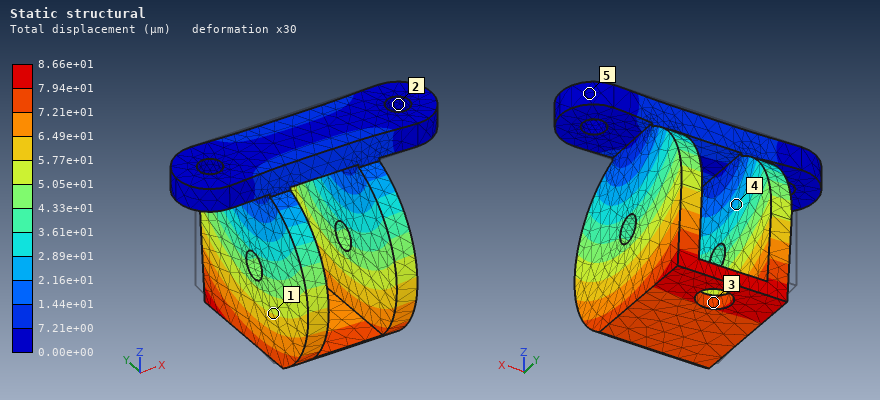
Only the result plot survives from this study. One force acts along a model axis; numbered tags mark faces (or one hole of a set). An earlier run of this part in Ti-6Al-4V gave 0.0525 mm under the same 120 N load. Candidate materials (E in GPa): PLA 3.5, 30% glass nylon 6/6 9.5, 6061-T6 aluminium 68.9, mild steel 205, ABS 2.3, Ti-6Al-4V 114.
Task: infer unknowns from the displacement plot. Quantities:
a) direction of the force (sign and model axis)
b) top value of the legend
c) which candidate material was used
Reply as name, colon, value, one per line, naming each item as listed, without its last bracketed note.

direction of the force: -Y
top value of the legend: 8.66e+01 µm
which candidate material was used: 6061-T6 aluminium
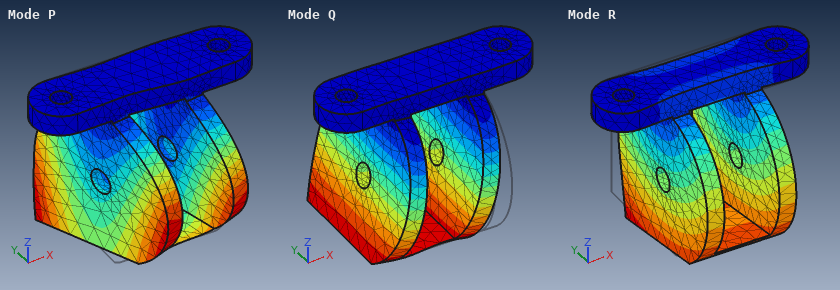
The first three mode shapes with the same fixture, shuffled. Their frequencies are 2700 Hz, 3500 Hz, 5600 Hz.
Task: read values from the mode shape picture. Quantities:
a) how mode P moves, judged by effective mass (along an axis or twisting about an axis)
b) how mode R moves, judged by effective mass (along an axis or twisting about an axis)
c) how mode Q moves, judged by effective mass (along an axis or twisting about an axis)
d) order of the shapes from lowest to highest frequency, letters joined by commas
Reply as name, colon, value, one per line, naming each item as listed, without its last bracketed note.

how mode P moves, judged by effective mass: twisting about Z
how mode R moves, judged by effective mass: along Y
how mode Q moves, judged by effective mass: along X
order of the shapes from lowest to highest frequency, letters joined by commas: R, Q, P
